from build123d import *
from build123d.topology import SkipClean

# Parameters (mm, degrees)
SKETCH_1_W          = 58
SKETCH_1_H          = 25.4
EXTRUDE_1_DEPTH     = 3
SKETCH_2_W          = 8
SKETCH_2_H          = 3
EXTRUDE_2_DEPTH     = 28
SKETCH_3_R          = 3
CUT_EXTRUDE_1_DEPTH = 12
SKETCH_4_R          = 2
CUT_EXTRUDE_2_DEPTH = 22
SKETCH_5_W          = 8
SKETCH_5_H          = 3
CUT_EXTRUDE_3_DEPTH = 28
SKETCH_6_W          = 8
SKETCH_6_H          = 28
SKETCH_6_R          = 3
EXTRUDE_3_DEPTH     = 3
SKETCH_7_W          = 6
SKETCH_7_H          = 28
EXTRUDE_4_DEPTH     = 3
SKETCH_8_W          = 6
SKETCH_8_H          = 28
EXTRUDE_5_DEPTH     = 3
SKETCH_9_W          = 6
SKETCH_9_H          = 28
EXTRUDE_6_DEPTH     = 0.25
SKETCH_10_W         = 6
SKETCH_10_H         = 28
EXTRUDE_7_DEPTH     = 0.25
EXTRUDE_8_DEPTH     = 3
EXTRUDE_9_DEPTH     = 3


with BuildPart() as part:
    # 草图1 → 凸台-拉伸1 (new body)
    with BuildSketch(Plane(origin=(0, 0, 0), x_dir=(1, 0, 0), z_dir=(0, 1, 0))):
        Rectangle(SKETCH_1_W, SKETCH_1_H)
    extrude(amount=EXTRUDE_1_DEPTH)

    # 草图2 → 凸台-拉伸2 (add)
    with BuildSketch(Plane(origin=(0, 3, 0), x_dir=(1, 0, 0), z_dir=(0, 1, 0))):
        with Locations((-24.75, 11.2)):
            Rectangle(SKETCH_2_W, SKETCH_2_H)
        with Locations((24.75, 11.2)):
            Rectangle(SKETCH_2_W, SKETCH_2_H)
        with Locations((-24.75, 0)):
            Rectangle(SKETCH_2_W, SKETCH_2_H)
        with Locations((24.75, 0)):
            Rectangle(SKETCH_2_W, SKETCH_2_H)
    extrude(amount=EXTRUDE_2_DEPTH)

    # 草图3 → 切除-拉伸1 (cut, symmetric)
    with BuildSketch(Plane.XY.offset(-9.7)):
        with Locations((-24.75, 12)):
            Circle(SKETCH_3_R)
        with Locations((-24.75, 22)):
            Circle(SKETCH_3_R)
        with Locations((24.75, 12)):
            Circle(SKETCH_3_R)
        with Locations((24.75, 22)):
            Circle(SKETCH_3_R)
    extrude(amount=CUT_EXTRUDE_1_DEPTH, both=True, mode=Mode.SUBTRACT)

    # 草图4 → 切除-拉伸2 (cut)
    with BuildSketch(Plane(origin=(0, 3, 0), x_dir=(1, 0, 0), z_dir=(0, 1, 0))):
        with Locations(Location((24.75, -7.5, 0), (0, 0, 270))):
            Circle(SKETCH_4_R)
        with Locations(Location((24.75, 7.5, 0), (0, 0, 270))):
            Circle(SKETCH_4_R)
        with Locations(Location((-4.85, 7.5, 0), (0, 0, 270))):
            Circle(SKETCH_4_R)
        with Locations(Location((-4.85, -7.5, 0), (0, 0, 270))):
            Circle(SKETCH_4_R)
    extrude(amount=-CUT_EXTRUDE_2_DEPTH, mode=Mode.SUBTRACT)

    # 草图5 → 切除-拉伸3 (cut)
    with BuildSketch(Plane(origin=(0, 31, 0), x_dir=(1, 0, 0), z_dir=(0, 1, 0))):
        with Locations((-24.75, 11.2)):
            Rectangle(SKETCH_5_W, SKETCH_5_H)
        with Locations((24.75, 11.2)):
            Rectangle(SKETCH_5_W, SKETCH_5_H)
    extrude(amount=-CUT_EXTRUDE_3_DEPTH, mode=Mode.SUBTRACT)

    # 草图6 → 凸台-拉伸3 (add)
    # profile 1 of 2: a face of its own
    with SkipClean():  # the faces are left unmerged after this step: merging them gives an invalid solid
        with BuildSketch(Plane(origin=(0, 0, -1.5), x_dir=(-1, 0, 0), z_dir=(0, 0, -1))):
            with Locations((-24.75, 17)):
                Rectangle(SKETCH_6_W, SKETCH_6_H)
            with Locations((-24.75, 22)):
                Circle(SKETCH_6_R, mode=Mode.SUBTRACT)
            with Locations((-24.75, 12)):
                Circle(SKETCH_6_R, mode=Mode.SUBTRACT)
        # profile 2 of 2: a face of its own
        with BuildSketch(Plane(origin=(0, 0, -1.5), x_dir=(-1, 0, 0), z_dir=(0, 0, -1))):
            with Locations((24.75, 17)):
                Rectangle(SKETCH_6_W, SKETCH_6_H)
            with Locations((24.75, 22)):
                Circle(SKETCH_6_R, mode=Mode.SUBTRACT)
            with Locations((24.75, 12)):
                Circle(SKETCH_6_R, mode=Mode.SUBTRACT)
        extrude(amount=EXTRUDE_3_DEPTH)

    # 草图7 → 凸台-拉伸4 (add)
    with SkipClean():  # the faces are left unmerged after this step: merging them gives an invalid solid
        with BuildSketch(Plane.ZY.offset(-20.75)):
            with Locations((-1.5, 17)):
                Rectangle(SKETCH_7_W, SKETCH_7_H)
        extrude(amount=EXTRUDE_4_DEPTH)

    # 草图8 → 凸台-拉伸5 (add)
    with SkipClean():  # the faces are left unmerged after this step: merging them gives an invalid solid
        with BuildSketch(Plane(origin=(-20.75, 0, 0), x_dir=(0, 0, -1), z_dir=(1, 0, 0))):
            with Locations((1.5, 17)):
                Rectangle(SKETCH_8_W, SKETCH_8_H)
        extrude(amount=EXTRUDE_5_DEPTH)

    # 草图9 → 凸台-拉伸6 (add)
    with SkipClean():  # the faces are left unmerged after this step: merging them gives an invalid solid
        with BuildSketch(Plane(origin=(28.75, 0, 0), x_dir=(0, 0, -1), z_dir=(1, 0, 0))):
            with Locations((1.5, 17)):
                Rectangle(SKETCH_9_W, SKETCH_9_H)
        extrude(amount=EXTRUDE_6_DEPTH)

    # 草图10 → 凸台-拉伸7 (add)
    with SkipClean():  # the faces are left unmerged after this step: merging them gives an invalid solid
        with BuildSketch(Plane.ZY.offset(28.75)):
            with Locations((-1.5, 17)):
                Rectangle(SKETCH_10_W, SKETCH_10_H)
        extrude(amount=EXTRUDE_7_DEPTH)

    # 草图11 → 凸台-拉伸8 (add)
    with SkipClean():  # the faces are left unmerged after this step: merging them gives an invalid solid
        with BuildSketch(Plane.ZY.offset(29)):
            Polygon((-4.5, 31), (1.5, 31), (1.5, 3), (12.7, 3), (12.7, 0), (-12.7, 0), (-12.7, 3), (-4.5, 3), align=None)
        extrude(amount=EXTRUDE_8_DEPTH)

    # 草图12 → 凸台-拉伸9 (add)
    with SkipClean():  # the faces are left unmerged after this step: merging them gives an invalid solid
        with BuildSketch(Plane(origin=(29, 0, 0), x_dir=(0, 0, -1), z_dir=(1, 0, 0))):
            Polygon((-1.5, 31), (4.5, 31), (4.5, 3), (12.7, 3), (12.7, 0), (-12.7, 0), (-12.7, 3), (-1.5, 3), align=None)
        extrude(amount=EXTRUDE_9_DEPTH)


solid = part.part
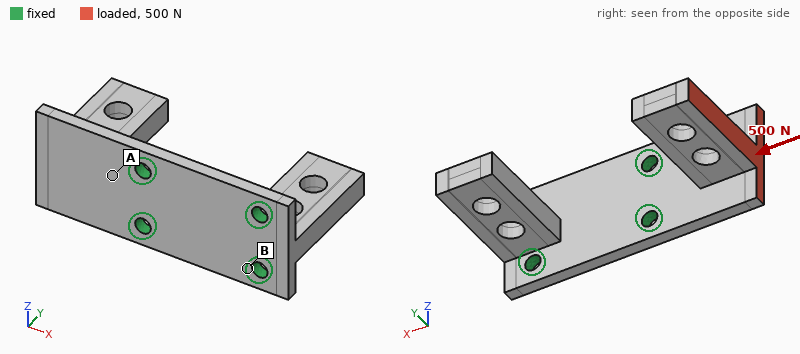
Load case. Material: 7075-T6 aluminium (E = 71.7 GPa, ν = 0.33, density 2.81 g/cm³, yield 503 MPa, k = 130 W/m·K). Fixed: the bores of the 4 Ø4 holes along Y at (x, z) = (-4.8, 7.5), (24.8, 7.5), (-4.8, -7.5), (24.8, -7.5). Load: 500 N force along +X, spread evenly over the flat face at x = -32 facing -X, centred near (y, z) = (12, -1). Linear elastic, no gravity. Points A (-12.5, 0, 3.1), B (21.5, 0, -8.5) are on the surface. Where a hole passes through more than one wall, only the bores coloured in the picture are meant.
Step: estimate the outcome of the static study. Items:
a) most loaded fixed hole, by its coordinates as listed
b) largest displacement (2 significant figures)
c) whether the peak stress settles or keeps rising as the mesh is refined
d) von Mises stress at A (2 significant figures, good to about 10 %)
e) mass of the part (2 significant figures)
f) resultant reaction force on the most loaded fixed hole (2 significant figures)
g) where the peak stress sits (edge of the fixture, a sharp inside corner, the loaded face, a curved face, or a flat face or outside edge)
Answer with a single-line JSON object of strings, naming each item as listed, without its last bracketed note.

{"most loaded fixed hole, by its coordinates as listed": "(-4.8, -7.5)", "largest displacement": "0.68 mm", "whether the peak stress settles or keeps rising as the mesh is refined": "keeps rising", "von Mises stress at A": "120 MPa", "mass of the part": "25 g", "resultant reaction force on the most loaded fixed hole": "270 N", "where the peak stress sits": "edge of the fixture"}
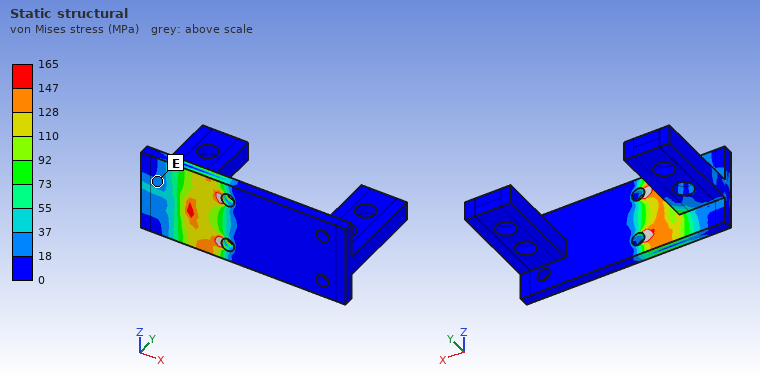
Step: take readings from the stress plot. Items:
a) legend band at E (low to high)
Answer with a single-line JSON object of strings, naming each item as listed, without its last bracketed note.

{"legend band at E": "18 to 37 MPa"}
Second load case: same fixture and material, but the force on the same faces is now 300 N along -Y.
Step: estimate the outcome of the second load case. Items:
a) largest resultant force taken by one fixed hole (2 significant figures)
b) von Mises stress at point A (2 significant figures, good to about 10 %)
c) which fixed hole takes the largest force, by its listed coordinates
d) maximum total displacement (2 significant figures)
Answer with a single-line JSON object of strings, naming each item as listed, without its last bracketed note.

{"largest resultant force taken by one fixed hole": "170 N", "von Mises stress at point A": "140 MPa", "which fixed hole takes the largest force, by its listed coordinates": "(-4.8, -7.5)", "maximum total displacement": "0.72 mm"}
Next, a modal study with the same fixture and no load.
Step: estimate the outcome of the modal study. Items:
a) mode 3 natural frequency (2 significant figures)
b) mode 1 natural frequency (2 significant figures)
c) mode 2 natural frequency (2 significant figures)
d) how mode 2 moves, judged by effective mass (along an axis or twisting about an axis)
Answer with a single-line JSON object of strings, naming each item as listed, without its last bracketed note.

{"mode 3 natural frequency": "4700 Hz", "mode 1 natural frequency": "1500 Hz", "mode 2 natural frequency": "2500 Hz", "how mode 2 moves, judged by effective mass": "along Z"}
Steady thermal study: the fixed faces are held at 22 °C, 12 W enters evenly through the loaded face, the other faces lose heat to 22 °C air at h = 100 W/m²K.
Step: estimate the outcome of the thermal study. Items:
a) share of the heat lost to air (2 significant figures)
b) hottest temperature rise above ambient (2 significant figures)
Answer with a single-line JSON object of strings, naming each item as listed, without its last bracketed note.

{"share of the heat lost to air": "33 %", "hottest temperature rise above ambient": "27 K"}
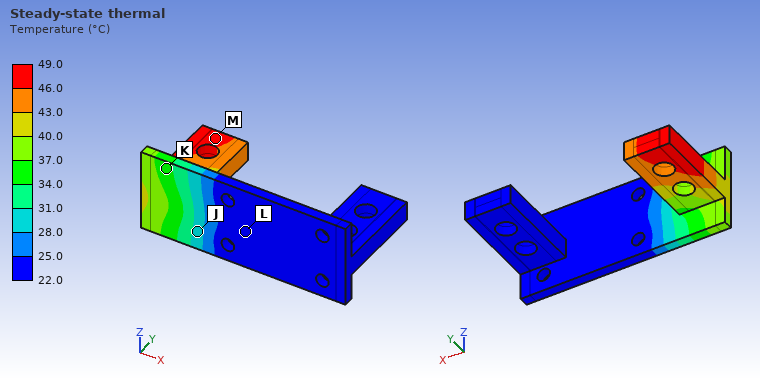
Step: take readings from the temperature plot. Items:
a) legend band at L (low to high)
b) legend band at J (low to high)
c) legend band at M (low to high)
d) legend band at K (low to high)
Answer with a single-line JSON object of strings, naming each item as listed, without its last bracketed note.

{"legend band at L": "22.0 to 25.0 °C", "legend band at J": "28.0 to 31.0 °C", "legend band at M": "46.0 to 49.0 °C", "legend band at K": "34.0 to 37.0 °C"}
